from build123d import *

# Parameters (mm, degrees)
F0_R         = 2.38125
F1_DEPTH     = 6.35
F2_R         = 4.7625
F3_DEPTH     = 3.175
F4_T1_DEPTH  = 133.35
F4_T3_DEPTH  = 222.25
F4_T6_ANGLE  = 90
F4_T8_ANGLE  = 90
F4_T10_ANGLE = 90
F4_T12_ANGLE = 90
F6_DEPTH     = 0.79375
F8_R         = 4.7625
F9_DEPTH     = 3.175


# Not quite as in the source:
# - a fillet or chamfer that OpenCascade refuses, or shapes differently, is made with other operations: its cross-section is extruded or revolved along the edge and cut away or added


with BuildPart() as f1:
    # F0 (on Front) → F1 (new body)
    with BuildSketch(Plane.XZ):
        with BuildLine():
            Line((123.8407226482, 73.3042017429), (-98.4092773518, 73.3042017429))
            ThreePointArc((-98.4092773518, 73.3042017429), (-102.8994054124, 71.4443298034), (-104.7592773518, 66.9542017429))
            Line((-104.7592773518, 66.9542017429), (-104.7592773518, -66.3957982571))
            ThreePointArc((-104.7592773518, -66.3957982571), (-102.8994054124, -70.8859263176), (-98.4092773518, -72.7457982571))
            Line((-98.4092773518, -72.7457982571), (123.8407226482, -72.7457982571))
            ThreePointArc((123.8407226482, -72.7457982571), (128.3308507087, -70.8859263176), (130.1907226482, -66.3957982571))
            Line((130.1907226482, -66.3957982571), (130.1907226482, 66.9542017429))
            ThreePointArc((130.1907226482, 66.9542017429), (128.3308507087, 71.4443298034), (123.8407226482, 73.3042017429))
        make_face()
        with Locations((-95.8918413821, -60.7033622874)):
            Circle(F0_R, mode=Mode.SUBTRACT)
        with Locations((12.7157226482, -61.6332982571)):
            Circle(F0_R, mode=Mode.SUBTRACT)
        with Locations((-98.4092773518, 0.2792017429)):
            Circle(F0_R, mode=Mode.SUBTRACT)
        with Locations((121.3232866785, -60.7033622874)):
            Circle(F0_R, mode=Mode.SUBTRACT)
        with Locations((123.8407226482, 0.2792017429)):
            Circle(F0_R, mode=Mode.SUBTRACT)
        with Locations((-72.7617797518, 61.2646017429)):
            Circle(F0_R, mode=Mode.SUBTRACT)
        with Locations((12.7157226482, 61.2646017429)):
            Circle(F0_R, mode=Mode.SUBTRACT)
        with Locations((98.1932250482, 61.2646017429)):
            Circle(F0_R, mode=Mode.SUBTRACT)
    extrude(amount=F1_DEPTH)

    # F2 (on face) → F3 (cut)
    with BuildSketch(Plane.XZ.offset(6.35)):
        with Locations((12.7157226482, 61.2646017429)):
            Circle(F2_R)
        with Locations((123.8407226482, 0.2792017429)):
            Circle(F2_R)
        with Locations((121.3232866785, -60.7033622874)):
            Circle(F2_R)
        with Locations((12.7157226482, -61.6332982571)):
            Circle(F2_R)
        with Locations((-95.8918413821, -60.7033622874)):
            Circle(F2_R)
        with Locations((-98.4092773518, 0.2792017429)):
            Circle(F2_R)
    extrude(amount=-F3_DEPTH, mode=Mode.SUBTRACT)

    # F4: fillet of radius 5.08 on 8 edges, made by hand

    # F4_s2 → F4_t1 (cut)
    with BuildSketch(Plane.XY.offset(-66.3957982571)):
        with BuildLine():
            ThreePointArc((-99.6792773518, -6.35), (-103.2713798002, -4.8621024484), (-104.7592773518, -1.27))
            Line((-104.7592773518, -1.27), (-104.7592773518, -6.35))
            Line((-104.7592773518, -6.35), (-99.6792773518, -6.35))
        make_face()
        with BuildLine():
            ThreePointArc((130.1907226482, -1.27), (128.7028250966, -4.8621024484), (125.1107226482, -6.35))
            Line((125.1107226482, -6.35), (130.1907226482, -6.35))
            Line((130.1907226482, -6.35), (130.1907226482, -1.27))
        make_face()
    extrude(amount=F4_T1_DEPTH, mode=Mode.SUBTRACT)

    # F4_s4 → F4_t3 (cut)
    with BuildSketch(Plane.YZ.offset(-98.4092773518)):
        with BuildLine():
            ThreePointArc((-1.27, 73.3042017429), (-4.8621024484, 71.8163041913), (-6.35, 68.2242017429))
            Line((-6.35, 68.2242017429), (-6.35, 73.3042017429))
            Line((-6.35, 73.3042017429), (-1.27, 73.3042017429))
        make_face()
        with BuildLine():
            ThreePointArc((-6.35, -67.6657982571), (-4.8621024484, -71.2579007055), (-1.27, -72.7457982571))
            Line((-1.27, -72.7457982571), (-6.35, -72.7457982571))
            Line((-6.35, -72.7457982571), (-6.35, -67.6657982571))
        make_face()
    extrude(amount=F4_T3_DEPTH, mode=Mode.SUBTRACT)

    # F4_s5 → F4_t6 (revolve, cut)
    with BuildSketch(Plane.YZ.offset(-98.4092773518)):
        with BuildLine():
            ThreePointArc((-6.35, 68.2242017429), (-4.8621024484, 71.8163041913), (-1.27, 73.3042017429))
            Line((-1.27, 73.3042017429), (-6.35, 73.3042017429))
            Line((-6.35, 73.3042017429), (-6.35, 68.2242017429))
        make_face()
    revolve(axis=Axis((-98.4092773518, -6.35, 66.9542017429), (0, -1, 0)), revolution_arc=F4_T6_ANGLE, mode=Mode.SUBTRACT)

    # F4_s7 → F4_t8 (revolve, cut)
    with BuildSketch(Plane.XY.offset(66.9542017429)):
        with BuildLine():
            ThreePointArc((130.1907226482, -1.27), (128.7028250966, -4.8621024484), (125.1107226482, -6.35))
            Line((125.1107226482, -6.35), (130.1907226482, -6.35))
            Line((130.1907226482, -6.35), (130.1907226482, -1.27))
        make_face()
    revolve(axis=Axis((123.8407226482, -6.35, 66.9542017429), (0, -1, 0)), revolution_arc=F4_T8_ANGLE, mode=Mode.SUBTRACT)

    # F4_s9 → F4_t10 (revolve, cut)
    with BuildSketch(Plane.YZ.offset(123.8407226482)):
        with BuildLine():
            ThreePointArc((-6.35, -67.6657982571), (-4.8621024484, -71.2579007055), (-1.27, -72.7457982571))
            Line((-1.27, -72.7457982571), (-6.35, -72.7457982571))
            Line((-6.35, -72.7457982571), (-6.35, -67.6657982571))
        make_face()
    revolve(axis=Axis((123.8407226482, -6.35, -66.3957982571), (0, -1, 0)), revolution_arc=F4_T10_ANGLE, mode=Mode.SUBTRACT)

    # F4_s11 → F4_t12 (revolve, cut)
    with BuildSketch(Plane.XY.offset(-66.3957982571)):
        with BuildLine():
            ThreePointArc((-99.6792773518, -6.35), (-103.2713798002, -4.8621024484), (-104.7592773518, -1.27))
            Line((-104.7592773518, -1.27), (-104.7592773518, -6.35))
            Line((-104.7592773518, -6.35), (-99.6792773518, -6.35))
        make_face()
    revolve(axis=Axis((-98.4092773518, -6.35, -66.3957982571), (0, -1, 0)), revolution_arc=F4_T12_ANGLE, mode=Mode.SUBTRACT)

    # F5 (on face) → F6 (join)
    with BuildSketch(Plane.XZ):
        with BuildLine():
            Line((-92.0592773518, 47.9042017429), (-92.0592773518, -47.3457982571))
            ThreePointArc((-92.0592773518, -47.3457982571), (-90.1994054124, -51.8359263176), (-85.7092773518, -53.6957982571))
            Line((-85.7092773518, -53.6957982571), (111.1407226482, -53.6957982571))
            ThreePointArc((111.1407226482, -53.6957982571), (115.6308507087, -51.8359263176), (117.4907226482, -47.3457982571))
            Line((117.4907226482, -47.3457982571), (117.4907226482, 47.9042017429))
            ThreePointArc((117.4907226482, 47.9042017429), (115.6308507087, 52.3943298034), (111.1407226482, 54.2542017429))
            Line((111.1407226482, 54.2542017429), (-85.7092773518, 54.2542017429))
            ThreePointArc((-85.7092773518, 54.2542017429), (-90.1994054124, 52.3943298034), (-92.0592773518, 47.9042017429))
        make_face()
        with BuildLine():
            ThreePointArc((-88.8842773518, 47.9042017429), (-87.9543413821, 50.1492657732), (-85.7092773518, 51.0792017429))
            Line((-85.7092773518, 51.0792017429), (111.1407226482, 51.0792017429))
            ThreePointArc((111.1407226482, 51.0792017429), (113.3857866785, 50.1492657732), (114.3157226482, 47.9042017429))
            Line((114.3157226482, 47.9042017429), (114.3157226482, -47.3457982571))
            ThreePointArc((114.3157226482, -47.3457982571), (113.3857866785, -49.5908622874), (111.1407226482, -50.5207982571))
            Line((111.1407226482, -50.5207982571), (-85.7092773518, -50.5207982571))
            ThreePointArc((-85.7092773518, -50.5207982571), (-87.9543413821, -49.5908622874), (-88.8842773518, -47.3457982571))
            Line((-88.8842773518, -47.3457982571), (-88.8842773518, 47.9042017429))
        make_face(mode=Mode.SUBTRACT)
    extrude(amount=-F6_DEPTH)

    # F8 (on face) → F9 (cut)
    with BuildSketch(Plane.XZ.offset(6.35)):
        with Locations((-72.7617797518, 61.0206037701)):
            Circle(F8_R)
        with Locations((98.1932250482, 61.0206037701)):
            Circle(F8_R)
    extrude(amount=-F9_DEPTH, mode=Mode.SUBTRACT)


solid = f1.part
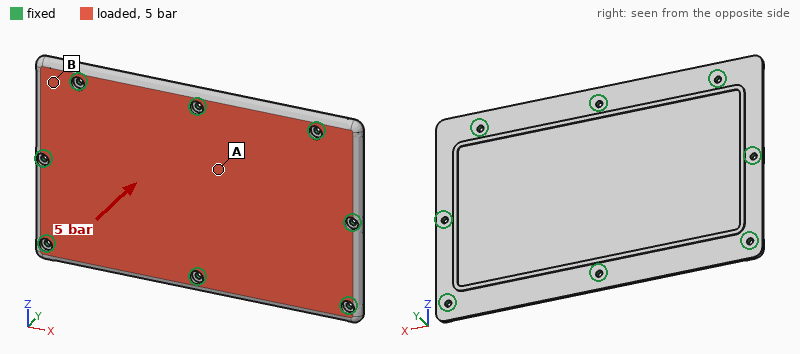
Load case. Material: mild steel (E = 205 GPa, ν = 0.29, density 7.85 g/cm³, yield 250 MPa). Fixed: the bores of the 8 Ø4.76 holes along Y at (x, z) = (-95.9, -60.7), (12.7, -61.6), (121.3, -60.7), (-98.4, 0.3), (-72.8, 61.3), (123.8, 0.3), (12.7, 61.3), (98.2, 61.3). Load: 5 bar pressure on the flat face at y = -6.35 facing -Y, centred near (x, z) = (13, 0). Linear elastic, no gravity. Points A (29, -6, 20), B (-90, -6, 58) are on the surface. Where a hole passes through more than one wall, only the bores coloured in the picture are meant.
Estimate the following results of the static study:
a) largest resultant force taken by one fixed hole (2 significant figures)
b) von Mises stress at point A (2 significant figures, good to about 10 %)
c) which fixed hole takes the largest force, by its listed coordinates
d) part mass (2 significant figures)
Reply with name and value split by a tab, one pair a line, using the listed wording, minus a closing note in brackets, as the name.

largest resultant force taken by one fixed hole	5.7 kN
von Mises stress at point A	59 MPa
which fixed hole takes the largest force, by its listed coordinates	(12.7, -61.6)
part mass	1.7 kg
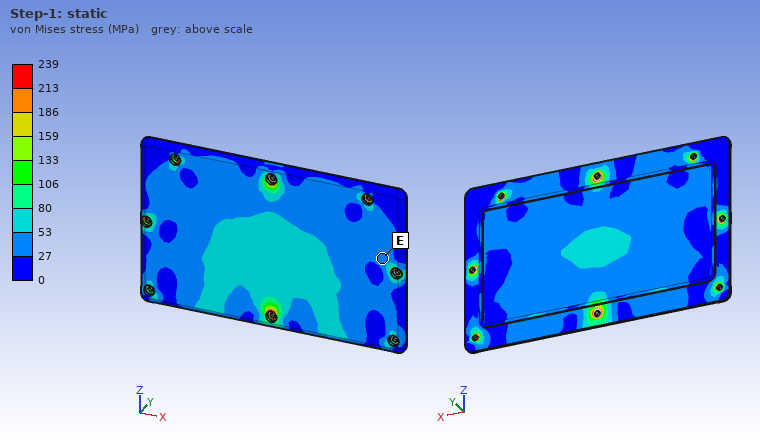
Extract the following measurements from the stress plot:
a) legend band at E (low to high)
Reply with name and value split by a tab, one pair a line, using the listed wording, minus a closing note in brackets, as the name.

legend band at E	27 to 53 MPa
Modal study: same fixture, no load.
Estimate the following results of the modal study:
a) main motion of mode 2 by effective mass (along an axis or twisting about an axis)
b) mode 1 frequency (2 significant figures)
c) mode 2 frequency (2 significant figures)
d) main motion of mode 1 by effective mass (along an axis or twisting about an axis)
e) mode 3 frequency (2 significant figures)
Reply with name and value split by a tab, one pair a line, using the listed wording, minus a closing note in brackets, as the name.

main motion of mode 2 by effective mass	twisting about Z
mode 1 frequency	1500 Hz
mode 2 frequency	1900 Hz
main motion of mode 1 by effective mass	along Y
mode 3 frequency	2800 Hz
